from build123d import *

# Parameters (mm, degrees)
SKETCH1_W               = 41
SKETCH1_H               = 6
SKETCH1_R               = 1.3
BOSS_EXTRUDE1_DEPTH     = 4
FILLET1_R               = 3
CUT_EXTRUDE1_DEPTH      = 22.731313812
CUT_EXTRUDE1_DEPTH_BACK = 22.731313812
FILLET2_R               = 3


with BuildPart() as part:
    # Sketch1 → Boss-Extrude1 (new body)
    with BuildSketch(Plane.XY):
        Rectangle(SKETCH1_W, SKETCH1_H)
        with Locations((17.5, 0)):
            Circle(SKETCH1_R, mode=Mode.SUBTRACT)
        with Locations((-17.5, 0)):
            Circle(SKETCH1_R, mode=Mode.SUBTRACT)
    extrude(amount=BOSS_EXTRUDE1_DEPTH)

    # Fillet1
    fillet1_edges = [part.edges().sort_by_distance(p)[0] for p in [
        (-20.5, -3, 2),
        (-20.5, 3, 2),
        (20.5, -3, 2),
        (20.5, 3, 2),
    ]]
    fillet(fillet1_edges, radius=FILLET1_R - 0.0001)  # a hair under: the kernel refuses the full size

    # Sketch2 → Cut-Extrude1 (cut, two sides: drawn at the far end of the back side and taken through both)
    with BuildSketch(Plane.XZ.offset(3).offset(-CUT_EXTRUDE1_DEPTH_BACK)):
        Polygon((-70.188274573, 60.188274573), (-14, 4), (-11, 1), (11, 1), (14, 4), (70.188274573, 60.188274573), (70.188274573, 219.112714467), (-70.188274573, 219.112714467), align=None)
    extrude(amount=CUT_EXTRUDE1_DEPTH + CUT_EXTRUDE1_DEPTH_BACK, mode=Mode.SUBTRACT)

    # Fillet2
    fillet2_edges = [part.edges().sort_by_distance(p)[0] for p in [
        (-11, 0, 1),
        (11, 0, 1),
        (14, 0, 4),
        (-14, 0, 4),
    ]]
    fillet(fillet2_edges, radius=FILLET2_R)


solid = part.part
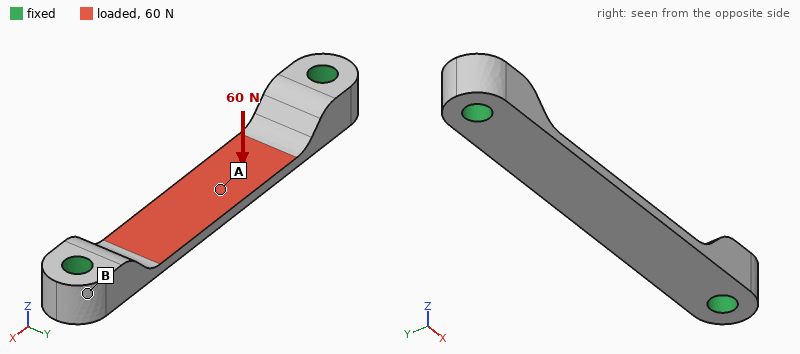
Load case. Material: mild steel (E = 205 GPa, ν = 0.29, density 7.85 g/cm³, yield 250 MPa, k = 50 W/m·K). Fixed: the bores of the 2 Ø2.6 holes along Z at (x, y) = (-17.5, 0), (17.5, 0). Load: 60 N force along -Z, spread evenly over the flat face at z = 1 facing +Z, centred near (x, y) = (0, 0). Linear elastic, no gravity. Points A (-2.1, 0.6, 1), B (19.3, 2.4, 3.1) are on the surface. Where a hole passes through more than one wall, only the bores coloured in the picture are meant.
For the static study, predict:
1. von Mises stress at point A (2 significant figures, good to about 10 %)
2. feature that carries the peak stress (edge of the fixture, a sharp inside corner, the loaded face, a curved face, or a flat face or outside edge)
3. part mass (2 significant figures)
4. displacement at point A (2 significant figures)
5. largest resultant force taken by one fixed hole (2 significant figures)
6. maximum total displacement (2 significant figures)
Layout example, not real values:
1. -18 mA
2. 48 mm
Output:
1. 50 MPa
2. a curved face
3. 3.6 g
4. 20 µm
5. 47 N
6. 22 µm
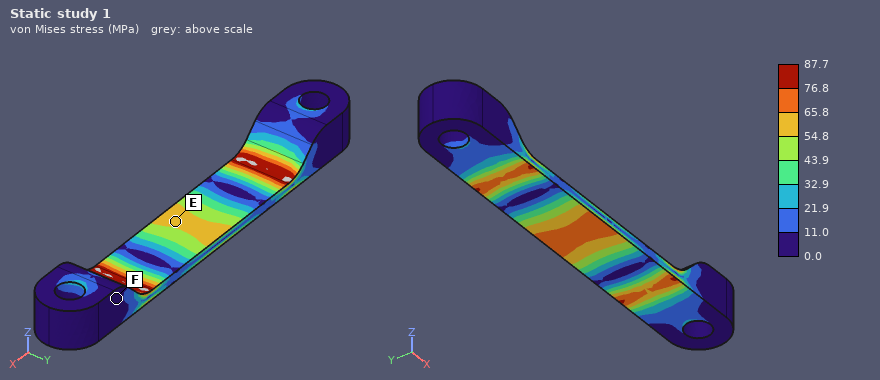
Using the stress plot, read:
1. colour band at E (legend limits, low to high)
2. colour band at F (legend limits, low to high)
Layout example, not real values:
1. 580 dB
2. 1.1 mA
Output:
1. 54.8 to 65.8 MPa
2. 0.0 to 11.0 MPa
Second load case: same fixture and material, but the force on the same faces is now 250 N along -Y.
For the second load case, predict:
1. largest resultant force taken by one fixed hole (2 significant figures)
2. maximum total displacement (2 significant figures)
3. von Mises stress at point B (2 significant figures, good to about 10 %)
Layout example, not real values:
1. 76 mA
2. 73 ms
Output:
1. 130 N
2. 13 µm
3. 7.1 MPa
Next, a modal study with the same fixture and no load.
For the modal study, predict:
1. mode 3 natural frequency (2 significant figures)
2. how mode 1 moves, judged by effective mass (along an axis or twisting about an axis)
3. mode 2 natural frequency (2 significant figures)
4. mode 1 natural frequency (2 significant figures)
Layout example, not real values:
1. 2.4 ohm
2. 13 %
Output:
1. 25 kHz
2. along Z
3. 24 kHz
4. 9900 Hz
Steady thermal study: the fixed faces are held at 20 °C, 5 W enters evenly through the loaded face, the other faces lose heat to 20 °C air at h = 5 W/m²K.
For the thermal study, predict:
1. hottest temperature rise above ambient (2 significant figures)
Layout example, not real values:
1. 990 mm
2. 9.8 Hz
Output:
1. 69 K
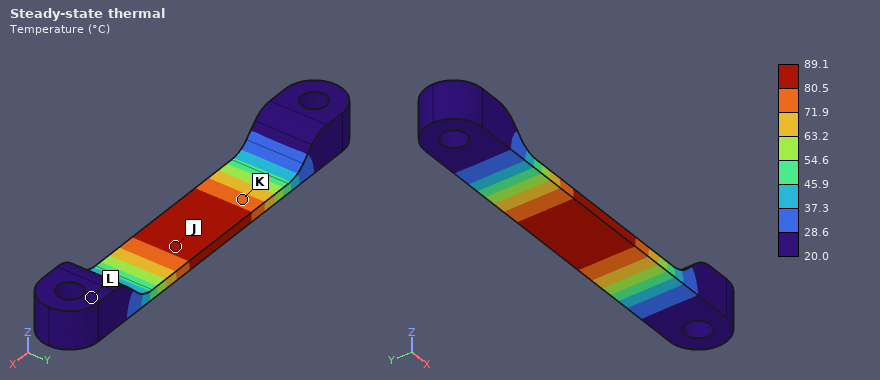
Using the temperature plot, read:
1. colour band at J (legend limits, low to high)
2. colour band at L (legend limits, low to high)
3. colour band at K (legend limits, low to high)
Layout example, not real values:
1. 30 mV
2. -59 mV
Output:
1. 80.5 to 89.1 °C
2. 20.0 to 28.6 °C
3. 71.9 to 80.5 °C
